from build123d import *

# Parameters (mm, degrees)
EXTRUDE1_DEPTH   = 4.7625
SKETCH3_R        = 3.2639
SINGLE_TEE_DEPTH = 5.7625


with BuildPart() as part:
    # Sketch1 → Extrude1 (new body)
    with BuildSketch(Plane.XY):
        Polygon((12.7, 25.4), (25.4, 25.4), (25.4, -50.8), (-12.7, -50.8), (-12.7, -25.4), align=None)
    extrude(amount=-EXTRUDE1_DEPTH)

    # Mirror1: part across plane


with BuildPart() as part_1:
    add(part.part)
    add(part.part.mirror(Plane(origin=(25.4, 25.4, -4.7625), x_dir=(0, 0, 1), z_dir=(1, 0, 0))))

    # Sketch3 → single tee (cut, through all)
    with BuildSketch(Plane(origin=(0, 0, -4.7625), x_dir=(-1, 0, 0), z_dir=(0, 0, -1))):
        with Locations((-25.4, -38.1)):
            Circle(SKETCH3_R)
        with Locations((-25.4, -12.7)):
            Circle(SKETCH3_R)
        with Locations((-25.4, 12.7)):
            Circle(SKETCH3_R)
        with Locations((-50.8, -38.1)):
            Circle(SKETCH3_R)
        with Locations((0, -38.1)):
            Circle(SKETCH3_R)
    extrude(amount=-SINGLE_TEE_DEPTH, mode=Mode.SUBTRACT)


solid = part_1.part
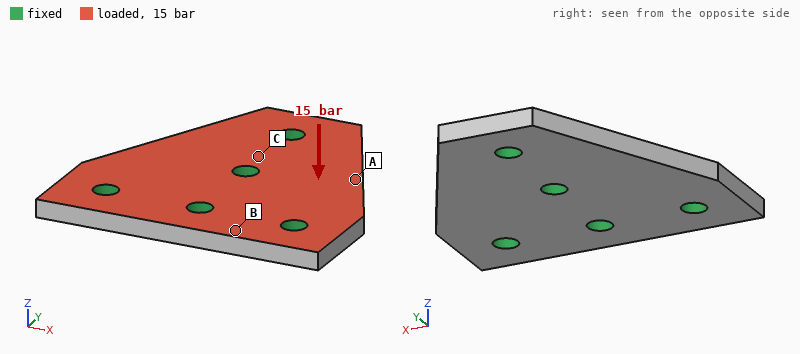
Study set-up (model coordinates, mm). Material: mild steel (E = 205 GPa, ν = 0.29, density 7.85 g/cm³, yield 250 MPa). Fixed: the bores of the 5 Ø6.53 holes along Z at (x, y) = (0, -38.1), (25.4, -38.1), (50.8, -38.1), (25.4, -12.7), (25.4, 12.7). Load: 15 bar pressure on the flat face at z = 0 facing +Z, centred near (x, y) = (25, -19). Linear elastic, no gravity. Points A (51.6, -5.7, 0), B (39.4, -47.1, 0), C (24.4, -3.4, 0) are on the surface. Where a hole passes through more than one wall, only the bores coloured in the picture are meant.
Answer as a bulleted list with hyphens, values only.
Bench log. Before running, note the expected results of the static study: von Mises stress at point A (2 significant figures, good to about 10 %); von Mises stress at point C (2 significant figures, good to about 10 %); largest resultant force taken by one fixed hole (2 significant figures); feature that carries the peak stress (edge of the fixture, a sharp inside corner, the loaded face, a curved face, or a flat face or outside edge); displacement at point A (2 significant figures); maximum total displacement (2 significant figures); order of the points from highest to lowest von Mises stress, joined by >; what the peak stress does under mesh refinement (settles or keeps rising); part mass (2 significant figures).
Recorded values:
- 26 MPa
- 47 MPa
- 1.6 kN
- edge of the fixture
- 21 µm
- 23 µm
- C > A > B
- keeps rising
- 160 g
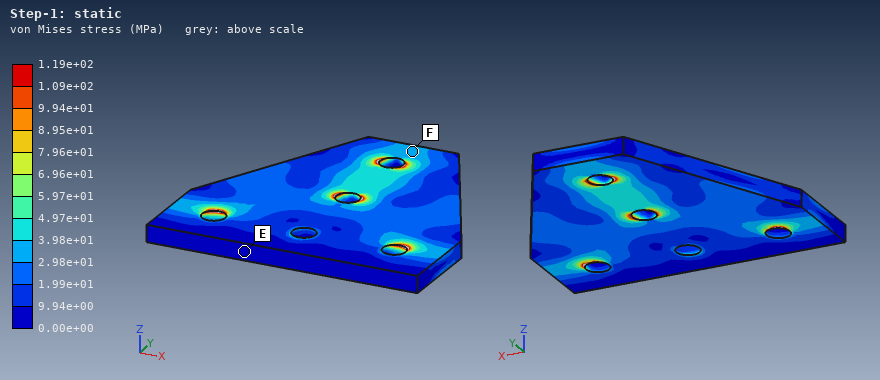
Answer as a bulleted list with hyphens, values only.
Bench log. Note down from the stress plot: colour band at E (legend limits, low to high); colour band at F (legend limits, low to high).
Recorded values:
- 0.00e+00 to 9.94e+00 MPa
- 2.98e+01 to 3.98e+01 MPa
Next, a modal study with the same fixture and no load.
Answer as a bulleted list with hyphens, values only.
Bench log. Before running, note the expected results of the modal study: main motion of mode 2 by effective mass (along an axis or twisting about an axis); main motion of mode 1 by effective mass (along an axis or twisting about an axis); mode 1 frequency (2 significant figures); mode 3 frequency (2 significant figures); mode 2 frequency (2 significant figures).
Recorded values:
- along Z
- twisting about Y
- 8500 Hz
- 16 kHz
- 8900 Hz
